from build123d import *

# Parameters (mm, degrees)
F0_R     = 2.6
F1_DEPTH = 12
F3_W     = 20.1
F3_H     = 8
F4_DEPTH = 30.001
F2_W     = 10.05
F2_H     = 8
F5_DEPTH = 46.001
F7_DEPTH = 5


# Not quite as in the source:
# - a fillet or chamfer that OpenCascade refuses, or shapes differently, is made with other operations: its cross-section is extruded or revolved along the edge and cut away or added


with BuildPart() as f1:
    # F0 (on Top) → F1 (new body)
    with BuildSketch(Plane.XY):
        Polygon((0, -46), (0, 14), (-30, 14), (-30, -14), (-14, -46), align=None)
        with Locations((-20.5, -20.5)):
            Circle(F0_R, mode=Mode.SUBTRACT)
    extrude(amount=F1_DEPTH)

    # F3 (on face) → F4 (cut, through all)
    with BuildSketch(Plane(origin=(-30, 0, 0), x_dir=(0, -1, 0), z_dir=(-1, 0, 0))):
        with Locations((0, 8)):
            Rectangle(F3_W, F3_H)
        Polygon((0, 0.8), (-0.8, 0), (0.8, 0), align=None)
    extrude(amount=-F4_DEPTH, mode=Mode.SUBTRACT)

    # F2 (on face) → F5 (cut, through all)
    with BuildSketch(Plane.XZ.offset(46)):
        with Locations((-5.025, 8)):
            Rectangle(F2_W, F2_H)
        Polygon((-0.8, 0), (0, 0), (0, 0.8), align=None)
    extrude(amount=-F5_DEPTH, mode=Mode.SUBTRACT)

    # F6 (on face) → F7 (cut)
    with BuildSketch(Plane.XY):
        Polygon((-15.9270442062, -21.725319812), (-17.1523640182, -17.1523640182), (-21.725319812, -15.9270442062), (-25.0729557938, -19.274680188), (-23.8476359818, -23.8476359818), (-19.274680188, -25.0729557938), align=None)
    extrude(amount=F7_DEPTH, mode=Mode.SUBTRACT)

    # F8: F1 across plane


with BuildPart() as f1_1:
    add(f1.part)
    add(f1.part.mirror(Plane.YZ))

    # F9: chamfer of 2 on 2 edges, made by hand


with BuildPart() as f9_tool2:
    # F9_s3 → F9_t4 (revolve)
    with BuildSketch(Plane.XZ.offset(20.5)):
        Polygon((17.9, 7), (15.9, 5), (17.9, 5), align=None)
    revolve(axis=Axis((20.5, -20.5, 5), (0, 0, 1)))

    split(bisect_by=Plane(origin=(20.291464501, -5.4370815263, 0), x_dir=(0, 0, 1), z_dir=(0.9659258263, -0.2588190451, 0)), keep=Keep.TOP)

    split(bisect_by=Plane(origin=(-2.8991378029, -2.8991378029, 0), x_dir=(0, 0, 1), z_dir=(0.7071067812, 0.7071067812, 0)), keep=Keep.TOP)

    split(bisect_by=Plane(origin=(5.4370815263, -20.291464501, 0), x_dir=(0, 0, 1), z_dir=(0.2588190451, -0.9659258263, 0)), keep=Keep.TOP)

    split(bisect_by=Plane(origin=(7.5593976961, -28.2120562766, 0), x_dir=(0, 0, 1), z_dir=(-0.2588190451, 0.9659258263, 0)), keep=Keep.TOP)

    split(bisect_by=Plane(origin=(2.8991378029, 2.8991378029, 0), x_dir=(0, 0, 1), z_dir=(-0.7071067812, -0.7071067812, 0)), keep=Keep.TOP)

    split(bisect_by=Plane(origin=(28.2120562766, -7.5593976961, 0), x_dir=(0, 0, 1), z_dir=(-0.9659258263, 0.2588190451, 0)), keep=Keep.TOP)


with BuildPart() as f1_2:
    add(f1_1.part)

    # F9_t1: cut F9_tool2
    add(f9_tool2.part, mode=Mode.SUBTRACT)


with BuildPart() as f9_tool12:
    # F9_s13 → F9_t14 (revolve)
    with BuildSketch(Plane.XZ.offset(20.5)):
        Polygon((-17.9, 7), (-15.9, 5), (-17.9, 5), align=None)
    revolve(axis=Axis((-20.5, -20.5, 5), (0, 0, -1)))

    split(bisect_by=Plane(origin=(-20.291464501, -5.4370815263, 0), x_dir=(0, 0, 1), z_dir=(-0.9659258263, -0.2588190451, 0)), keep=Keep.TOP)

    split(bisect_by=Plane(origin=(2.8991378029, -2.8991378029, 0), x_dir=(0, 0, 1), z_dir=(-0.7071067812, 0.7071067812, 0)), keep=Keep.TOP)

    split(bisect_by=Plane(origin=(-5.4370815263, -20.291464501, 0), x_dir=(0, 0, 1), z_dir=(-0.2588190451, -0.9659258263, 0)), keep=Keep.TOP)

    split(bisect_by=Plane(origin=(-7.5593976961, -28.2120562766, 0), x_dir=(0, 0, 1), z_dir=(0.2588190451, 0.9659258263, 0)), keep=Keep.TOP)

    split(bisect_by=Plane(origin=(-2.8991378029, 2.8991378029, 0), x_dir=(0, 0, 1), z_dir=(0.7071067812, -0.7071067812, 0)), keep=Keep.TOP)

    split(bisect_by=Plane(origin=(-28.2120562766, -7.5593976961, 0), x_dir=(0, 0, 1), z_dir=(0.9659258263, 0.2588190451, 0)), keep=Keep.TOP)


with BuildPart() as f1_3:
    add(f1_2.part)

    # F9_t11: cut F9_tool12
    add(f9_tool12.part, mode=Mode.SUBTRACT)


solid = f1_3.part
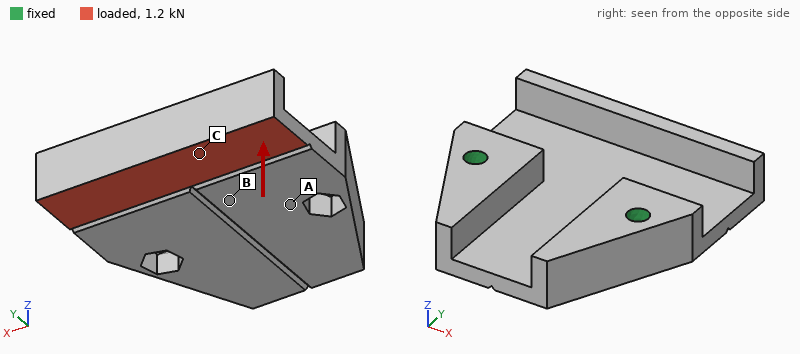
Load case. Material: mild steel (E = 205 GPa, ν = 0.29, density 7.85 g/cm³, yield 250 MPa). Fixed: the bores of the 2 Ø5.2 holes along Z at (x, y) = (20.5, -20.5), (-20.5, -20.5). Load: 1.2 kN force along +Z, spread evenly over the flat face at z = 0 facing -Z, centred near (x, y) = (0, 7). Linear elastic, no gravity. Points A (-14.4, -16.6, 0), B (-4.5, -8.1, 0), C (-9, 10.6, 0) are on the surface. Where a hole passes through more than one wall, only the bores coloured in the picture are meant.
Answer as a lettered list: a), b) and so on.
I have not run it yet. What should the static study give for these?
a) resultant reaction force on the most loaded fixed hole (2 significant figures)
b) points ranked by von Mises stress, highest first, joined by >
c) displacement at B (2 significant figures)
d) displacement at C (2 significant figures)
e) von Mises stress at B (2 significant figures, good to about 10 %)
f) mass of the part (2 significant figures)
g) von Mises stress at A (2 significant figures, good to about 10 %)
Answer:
a) 650 N
b) B > A > C
c) 0.019 mm
d) 0.089 mm
e) 90 MPa
f) 160 g
g) 47 MPa
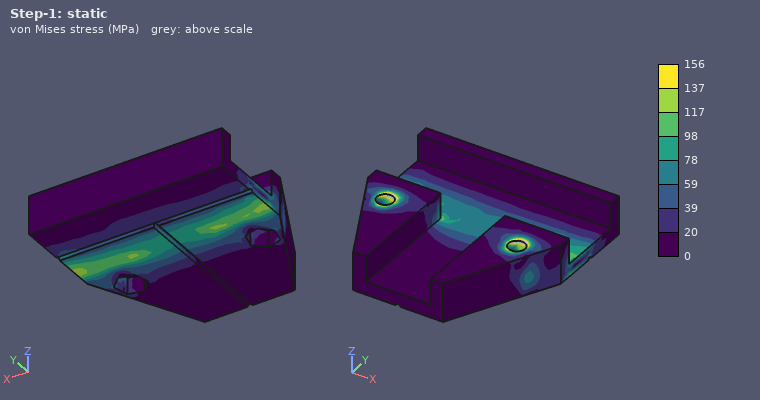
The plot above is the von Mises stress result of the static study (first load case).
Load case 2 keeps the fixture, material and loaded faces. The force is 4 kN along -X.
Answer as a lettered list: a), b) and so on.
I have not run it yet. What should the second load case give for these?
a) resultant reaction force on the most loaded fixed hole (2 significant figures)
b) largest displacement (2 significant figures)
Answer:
a) 3.1 kN
b) 21 µm
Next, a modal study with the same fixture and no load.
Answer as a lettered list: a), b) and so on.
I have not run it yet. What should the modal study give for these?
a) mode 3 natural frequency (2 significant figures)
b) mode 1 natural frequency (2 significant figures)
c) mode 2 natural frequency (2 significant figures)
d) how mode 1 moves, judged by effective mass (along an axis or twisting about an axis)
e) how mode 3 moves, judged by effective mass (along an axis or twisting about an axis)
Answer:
a) 7700 Hz
b) 2700 Hz
c) 4600 Hz
d) along Z
e) along Y
